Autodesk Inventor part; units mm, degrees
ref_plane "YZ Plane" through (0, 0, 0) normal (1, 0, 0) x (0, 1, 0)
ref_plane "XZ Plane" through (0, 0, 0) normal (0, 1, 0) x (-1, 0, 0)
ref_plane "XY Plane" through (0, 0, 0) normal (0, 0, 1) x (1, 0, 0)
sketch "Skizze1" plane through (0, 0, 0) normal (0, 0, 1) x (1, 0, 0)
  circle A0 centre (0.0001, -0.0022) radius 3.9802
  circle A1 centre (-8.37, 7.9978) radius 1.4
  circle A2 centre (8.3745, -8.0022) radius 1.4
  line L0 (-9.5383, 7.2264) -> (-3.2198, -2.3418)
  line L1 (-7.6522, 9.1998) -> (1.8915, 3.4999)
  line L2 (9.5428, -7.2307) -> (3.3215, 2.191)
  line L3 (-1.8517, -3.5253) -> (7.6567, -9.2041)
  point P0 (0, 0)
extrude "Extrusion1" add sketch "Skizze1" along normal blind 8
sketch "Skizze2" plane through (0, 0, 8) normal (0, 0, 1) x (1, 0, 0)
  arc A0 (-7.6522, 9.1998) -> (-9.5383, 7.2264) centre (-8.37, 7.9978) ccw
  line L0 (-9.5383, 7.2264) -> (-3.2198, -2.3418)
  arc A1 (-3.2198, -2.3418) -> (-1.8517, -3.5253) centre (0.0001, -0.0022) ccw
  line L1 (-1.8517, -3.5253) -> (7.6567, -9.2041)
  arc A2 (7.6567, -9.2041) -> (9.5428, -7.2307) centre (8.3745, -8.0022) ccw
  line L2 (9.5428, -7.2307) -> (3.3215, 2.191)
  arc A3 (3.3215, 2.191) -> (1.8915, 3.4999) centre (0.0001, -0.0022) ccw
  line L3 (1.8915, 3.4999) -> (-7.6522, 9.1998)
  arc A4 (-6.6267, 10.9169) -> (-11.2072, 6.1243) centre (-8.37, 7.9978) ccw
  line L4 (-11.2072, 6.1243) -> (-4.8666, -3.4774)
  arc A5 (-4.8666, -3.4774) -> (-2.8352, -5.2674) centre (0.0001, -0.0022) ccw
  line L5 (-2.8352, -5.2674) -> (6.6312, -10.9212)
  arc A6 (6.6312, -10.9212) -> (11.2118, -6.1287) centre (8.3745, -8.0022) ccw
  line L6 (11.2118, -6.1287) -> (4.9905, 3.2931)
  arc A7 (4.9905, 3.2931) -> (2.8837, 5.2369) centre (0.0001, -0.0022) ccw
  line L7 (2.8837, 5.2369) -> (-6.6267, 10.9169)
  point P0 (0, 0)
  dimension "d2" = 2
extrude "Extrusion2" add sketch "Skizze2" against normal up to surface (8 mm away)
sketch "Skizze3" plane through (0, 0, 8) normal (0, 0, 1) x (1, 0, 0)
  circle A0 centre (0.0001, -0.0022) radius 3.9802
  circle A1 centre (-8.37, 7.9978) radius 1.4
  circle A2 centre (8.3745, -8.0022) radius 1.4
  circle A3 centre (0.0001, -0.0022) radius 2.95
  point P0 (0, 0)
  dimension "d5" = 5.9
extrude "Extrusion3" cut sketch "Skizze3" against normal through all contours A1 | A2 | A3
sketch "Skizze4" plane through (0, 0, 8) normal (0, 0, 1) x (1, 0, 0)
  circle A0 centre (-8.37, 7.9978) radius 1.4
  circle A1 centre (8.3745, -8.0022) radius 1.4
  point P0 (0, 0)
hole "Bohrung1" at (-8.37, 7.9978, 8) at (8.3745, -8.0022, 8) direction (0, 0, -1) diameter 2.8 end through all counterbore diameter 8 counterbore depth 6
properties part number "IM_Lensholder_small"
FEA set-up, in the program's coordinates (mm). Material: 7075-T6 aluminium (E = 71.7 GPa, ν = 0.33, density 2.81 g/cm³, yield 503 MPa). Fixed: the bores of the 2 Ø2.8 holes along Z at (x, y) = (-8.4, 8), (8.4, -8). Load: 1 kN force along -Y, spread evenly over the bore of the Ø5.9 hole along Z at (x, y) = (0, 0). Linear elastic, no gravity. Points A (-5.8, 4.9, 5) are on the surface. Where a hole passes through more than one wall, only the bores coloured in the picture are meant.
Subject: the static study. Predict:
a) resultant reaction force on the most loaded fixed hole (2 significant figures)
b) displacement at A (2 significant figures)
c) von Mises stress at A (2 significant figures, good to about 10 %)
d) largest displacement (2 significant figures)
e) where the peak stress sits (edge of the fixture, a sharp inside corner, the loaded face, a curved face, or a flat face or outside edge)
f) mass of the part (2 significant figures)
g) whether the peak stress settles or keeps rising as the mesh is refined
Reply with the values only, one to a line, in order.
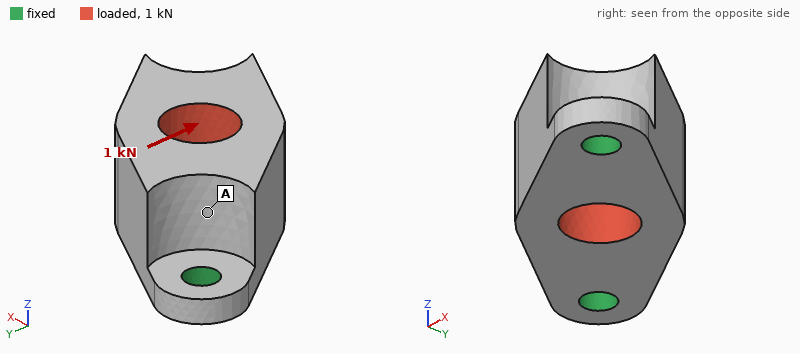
510 N
22 µm
31 MPa
44 µm
edge of the fixture
3.7 g
keeps rising
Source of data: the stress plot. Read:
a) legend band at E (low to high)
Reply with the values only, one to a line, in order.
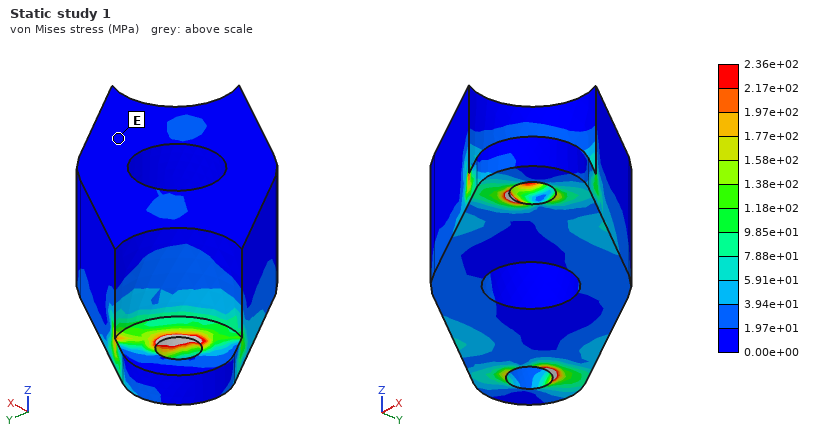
0.00e+00 to 1.97e+01 MPa
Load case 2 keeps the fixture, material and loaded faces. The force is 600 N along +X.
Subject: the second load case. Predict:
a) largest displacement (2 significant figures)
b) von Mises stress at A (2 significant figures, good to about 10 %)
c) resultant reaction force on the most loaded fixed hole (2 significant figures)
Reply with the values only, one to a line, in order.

25 µm
18 MPa
310 N
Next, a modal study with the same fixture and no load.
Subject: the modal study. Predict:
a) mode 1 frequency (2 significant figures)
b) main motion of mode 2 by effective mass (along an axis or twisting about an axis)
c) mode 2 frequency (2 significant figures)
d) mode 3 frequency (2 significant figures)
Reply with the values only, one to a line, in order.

12 kHz
along Z
25 kHz
40 kHz
